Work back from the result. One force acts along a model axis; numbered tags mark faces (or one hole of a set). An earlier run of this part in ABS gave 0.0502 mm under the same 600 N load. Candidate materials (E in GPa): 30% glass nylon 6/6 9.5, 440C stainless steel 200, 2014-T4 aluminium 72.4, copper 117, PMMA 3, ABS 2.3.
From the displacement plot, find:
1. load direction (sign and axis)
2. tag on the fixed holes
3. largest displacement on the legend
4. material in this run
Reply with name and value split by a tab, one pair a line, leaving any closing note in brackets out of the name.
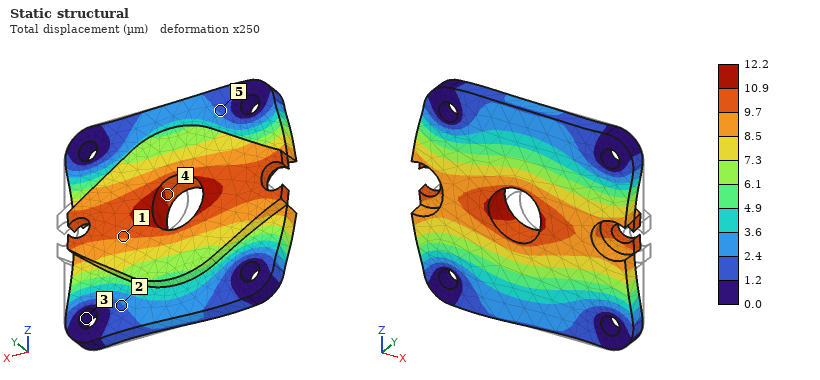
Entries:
load direction	-X
tag on the fixed holes	3
largest displacement on the legend	12.2 µm
material in this run	30% glass nylon 6/6
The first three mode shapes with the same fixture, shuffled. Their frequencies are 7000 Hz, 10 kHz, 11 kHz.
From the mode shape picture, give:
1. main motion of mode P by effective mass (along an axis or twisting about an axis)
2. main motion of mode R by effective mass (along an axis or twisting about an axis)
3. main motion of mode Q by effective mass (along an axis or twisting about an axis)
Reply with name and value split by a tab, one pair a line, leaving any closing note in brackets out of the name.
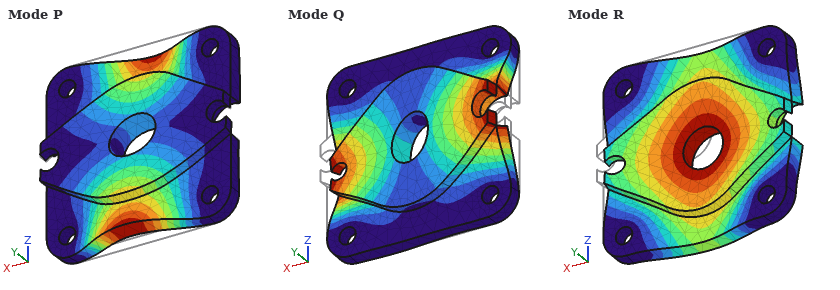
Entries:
main motion of mode P by effective mass	twisting about X
main motion of mode R by effective mass	along Y
main motion of mode Q by effective mass	twisting about Z
